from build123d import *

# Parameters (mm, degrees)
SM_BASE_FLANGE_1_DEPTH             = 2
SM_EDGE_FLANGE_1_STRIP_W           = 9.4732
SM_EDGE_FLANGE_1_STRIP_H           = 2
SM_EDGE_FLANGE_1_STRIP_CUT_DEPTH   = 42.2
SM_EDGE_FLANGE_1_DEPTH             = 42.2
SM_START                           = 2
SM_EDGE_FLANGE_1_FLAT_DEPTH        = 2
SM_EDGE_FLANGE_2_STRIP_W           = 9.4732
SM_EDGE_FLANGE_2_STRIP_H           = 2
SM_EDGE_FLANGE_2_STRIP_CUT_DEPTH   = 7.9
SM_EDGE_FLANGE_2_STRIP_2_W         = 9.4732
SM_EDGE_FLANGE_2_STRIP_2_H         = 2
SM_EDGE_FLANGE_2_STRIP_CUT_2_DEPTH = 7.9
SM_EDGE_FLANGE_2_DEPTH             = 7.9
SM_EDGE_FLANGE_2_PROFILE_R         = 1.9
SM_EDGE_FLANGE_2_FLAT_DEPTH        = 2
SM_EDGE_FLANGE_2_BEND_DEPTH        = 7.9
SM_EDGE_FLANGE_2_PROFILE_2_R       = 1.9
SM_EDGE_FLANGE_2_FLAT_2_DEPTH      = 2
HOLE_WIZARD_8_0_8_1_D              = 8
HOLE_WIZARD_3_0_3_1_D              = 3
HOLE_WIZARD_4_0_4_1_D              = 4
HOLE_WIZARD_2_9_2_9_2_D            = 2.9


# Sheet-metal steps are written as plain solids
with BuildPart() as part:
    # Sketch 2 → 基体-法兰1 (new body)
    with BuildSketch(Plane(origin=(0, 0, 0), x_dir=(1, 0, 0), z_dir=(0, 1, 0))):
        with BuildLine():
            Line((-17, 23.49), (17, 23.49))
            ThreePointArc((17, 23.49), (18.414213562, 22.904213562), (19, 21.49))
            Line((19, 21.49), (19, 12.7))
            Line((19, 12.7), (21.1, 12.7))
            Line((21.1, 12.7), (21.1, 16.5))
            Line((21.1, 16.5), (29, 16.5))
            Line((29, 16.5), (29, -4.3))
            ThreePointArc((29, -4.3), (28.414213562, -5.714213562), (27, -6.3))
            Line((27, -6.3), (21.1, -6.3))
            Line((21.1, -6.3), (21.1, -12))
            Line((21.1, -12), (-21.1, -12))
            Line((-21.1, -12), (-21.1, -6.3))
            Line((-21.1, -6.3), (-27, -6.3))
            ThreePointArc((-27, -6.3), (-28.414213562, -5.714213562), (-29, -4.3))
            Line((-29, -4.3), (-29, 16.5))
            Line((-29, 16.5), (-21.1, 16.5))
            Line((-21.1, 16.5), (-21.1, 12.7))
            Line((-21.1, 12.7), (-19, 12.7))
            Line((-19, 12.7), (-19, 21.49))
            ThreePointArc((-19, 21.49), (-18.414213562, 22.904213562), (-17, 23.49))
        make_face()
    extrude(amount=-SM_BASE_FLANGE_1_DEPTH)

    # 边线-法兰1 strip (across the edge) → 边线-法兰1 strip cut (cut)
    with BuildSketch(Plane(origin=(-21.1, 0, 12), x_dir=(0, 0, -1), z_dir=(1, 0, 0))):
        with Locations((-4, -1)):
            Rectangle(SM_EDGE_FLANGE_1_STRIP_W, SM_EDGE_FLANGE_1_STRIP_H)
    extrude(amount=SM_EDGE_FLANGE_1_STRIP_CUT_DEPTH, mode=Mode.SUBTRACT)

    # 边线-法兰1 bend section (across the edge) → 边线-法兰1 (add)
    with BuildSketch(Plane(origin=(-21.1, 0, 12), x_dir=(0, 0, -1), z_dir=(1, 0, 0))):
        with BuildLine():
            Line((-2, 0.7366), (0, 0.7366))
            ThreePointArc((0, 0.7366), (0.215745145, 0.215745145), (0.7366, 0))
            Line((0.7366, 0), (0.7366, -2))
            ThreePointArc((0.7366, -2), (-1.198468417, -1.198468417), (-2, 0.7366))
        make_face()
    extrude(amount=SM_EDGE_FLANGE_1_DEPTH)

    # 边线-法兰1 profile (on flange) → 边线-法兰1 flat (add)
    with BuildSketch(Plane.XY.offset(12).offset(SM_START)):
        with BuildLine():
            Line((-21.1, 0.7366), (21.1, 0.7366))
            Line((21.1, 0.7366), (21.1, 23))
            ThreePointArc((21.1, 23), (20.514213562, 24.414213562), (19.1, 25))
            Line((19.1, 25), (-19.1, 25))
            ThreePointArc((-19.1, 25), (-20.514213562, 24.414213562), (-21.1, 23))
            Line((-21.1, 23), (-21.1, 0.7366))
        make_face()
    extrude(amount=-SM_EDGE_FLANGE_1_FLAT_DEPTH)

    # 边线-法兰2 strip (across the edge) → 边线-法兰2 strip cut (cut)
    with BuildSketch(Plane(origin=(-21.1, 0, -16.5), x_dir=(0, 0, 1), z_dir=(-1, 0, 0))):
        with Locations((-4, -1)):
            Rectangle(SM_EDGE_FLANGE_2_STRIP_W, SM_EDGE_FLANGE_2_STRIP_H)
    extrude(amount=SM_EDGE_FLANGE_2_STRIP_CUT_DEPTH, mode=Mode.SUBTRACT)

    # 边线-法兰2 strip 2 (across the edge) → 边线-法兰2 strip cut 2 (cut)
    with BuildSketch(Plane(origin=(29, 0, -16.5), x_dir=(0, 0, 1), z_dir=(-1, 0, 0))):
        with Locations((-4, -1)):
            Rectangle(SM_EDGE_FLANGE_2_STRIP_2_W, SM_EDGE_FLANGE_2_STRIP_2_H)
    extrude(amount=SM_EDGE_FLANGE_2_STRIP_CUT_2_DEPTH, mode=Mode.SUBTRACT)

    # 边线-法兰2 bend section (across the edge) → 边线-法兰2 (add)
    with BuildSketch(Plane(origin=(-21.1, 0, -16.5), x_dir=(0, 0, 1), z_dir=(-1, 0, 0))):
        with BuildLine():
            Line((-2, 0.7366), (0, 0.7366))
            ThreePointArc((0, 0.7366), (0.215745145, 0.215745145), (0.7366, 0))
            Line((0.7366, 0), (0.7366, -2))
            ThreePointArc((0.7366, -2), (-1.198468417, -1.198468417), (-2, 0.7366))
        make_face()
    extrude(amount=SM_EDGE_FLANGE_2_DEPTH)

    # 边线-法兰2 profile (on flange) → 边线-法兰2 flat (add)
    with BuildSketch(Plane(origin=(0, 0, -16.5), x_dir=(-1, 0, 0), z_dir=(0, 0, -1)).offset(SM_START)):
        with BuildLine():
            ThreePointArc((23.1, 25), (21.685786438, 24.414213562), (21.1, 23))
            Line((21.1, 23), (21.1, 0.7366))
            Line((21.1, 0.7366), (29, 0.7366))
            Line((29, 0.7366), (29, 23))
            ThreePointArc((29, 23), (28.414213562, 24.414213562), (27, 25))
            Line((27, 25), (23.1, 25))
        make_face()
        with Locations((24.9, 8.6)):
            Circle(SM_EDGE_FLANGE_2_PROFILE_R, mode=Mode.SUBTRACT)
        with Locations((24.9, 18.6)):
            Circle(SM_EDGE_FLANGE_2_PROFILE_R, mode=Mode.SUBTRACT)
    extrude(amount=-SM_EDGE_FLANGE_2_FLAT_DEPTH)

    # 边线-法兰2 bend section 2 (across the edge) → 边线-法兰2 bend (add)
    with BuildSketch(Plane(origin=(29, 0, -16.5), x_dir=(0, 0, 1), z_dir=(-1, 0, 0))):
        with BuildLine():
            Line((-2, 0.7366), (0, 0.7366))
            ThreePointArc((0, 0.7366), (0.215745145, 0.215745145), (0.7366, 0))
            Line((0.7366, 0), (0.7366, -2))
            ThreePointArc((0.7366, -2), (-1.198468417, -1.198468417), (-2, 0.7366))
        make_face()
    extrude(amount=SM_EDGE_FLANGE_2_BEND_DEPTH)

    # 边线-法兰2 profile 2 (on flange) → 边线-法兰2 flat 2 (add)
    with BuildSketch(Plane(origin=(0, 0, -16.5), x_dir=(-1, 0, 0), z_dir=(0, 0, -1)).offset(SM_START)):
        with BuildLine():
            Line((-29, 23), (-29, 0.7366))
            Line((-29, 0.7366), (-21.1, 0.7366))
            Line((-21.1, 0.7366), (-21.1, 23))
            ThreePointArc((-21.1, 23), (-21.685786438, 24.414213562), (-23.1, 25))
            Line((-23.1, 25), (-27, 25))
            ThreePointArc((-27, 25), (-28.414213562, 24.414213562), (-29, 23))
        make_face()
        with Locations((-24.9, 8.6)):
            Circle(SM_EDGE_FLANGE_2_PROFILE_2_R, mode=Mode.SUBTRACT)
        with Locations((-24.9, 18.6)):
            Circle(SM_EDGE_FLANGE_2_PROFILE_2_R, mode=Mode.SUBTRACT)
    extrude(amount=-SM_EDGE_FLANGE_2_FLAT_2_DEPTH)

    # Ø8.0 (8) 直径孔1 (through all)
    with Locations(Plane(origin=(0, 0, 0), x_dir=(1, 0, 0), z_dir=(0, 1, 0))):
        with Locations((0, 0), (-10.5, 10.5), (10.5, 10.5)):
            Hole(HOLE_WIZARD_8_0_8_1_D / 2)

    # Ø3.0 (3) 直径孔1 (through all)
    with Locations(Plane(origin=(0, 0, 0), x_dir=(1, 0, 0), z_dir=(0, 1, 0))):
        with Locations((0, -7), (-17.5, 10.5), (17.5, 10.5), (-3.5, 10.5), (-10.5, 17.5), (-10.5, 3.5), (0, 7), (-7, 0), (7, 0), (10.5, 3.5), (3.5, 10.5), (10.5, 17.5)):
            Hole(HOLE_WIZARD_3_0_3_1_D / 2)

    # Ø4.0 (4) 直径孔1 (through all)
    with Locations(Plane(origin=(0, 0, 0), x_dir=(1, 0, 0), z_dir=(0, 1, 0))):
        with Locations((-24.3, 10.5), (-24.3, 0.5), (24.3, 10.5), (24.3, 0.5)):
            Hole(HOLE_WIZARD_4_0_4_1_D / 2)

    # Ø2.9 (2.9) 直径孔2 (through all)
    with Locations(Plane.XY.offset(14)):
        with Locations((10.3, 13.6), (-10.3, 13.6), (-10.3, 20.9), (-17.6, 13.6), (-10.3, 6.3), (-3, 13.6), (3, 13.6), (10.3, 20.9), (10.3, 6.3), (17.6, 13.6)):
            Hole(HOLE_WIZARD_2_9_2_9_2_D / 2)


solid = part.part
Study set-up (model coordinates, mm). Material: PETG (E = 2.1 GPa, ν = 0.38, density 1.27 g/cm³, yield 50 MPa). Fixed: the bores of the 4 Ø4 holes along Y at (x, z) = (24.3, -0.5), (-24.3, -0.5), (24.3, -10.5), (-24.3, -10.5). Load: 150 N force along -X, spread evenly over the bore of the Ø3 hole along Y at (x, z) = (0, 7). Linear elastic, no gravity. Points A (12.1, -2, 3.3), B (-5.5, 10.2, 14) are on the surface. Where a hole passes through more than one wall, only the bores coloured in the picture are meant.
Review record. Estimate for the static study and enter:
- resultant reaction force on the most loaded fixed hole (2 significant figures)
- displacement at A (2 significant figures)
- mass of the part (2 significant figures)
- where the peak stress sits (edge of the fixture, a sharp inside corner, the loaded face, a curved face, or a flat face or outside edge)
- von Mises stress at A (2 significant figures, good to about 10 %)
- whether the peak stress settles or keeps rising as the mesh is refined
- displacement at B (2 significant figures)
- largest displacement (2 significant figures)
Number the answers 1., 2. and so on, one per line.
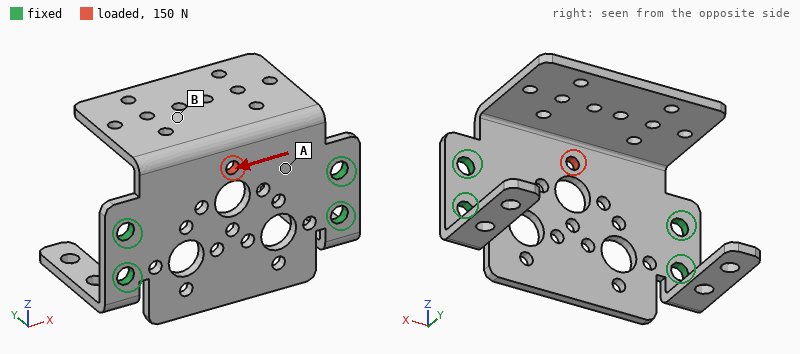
1. 67 N
2. 22 µm
3. 7.4 g
4. a sharp inside corner
5. 4.0 MPa
6. keeps rising
7. 33 µm
8. 54 µm
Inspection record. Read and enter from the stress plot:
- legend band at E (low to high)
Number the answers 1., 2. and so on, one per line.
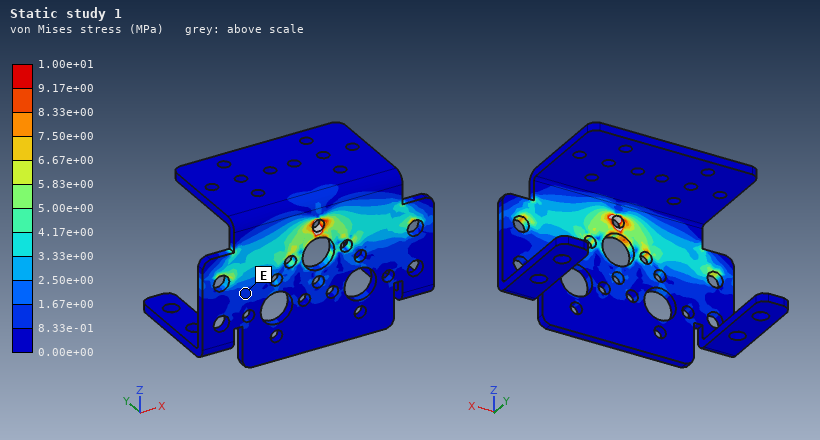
1. 8.33e-01 to 1.67e+00 MPa
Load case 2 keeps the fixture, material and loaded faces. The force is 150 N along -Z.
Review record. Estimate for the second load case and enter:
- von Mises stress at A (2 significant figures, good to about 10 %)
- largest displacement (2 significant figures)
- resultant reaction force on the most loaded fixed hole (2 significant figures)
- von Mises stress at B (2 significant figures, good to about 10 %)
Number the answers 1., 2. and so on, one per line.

1. 3.4 MPa
2. 0.12 mm
3. 48 N
4. 0.80 MPa
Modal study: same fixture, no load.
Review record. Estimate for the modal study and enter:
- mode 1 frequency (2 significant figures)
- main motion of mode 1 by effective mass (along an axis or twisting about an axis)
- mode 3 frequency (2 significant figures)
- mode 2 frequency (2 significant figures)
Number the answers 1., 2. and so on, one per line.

1. 320 Hz
2. along Z
3. 490 Hz
4. 490 Hz
